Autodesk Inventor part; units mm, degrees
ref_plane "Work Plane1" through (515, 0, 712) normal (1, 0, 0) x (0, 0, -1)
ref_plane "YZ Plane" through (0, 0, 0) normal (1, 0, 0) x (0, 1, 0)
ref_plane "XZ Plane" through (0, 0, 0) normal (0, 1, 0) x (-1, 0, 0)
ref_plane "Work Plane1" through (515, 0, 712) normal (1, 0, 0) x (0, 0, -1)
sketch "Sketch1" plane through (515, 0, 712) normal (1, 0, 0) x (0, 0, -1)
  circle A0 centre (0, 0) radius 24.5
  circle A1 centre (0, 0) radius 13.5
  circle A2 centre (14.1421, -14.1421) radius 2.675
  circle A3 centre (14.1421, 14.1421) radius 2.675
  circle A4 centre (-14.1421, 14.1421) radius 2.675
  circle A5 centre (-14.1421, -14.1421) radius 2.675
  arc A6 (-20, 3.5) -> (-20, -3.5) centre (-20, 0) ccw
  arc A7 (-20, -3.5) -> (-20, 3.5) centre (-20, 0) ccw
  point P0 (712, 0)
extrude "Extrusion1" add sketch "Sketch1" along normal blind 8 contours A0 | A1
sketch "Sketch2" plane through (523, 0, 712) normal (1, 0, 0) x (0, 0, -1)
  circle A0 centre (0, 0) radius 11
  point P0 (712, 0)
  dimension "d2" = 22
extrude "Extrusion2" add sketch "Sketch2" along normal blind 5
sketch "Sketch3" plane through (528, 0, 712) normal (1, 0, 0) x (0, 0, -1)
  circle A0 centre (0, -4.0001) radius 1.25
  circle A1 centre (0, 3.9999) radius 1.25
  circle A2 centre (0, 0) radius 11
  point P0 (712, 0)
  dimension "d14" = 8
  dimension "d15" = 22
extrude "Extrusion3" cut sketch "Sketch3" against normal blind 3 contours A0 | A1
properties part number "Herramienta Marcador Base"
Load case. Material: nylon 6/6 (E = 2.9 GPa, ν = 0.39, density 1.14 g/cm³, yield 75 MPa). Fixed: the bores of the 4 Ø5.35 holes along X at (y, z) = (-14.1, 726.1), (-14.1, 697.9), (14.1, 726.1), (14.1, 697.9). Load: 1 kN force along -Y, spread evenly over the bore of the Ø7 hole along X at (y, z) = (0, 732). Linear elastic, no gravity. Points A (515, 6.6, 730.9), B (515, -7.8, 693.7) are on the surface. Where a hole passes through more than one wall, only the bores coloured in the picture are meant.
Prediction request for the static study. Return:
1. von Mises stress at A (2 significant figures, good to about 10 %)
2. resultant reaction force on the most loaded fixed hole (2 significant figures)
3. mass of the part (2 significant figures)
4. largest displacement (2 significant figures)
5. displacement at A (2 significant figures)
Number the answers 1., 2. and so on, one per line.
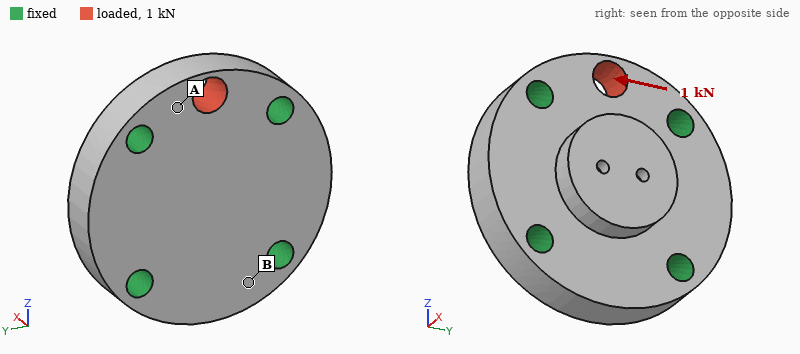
1. 6.7 MPa
2. 520 N
3. 18 g
4. 62 µm
5. 20 µm
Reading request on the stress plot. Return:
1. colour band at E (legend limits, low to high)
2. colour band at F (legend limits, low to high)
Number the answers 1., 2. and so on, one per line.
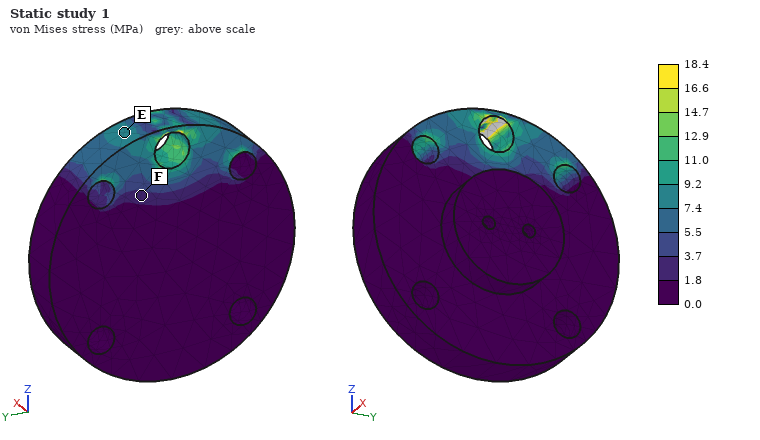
1. 7.4 to 9.2 MPa
2. 1.8 to 3.7 MPa
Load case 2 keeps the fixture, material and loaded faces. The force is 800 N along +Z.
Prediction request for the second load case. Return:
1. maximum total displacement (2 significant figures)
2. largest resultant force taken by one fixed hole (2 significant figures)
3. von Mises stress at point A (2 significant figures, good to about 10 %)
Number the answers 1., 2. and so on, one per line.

1. 85 µm
2. 290 N
3. 6.5 MPa
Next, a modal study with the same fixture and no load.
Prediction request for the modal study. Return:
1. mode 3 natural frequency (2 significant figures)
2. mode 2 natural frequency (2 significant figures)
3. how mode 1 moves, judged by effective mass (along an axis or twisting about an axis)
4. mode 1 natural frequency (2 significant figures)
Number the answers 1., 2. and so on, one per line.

1. 11 kHz
2. 11 kHz
3. along X
4. 9300 Hz
